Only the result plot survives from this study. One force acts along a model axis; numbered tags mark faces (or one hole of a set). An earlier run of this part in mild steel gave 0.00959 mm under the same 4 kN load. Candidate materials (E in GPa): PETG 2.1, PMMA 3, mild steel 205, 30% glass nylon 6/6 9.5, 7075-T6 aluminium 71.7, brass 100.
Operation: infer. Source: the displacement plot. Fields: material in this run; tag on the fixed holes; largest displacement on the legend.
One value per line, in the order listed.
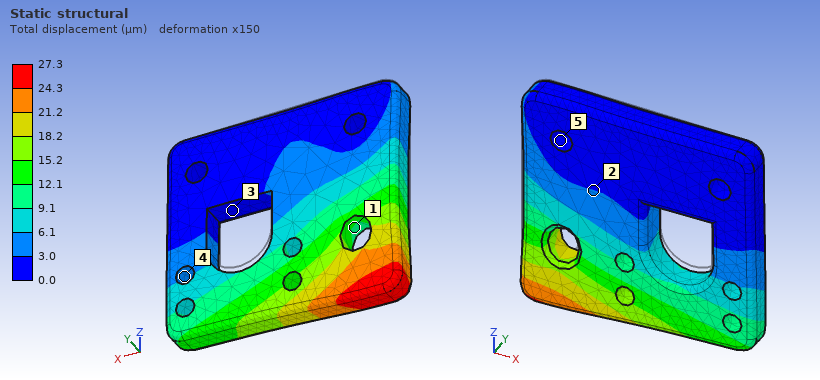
7075-T6 aluminium
5
27.3 µm
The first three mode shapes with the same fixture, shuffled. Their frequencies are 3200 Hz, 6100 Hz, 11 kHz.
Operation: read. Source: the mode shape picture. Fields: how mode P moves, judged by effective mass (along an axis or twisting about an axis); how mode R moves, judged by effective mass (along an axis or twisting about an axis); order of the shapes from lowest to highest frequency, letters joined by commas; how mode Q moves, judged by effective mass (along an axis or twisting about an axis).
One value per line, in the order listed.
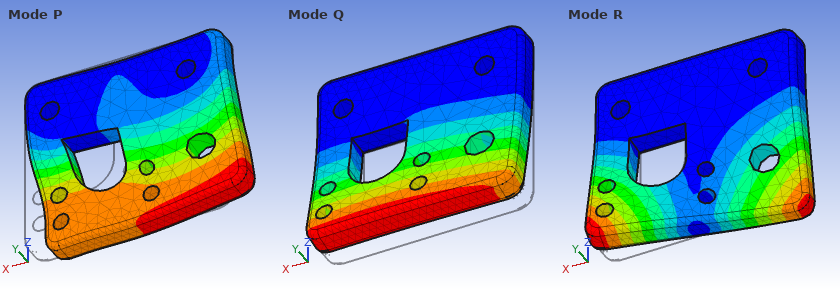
along X
twisting about Z
Q, R, P
along Y
